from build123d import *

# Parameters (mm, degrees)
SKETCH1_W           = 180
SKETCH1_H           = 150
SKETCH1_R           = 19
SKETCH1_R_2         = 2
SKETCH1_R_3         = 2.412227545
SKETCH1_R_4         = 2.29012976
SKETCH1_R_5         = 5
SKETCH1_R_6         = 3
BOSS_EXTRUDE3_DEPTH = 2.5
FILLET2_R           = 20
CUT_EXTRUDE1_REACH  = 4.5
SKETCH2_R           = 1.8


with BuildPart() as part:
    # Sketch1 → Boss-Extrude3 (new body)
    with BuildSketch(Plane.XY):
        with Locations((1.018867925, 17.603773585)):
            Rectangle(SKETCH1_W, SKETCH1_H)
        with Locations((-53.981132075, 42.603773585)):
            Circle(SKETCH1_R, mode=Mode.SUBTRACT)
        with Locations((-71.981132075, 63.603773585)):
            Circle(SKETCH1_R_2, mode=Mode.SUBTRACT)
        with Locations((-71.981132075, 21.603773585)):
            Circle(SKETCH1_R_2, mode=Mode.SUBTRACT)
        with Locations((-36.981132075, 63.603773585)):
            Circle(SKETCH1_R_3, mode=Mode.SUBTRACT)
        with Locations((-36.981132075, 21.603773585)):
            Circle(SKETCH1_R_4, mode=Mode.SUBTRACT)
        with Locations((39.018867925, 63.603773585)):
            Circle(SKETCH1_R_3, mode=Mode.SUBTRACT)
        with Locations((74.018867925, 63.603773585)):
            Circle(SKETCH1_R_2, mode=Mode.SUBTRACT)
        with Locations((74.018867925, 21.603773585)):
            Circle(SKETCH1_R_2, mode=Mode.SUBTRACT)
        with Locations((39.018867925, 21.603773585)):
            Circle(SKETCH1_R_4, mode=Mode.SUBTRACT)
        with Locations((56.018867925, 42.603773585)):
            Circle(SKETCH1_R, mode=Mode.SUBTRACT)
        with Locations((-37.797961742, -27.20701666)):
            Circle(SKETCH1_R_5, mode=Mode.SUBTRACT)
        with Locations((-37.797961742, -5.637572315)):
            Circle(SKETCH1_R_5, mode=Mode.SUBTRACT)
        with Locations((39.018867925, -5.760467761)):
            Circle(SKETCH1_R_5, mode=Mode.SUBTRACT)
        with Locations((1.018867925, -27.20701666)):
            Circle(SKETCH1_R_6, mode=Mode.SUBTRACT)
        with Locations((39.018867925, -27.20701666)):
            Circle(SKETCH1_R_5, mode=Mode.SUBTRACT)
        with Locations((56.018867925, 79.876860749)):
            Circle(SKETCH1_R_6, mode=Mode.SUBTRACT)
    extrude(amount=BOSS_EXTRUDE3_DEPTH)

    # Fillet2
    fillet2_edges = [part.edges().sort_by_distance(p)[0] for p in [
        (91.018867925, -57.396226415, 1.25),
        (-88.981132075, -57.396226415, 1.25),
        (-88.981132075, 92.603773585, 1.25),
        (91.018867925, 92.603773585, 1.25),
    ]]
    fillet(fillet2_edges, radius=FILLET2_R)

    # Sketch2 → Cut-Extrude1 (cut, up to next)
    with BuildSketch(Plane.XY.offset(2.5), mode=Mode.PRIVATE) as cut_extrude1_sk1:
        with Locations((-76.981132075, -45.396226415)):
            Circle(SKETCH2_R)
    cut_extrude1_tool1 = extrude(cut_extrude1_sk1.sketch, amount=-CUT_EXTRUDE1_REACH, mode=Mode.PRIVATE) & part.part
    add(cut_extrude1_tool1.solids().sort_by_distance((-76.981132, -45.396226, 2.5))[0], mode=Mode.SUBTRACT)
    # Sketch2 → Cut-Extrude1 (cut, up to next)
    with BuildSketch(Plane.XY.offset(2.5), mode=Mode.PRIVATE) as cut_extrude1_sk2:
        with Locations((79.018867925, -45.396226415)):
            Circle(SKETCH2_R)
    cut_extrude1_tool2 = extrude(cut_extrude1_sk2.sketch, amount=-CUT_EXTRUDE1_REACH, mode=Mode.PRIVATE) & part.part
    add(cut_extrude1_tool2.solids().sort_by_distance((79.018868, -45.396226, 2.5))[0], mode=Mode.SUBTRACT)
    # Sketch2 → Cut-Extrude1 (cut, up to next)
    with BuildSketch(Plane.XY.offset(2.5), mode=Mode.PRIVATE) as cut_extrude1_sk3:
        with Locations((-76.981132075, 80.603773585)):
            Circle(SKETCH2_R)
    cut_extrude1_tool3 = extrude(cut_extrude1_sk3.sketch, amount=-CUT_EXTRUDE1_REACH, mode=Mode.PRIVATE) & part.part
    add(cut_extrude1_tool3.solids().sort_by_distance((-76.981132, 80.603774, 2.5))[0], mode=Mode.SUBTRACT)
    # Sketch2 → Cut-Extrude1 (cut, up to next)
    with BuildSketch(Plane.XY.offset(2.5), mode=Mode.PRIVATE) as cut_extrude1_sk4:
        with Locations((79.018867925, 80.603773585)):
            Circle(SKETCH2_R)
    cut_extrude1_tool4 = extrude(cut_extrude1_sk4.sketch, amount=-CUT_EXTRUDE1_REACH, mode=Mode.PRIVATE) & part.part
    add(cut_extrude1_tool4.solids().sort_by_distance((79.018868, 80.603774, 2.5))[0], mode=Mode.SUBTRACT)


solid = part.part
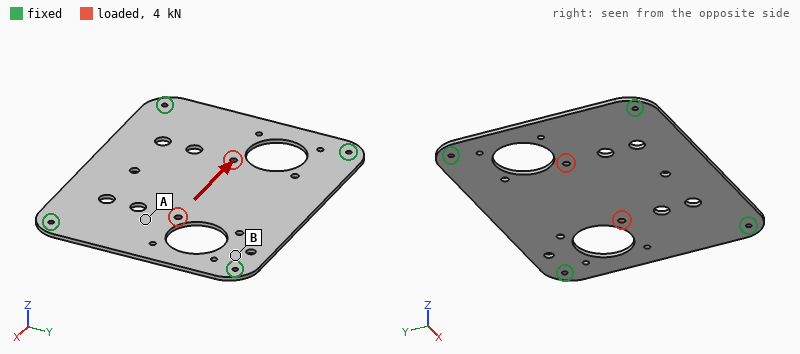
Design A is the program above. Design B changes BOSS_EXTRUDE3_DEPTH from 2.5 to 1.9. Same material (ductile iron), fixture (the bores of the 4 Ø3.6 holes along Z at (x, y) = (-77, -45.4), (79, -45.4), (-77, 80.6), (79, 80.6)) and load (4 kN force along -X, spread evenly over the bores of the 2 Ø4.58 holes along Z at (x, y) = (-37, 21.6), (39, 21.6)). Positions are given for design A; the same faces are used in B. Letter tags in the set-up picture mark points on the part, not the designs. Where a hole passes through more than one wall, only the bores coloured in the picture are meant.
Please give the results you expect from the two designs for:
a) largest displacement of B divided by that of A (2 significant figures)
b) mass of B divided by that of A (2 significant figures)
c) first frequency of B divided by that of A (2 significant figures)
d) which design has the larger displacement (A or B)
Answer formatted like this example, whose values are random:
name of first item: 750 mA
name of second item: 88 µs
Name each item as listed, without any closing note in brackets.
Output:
largest displacement of B divided by that of A: 1.3
mass of B divided by that of A: 0.76
first frequency of B divided by that of A: 0.77
which design has the larger displacement: B
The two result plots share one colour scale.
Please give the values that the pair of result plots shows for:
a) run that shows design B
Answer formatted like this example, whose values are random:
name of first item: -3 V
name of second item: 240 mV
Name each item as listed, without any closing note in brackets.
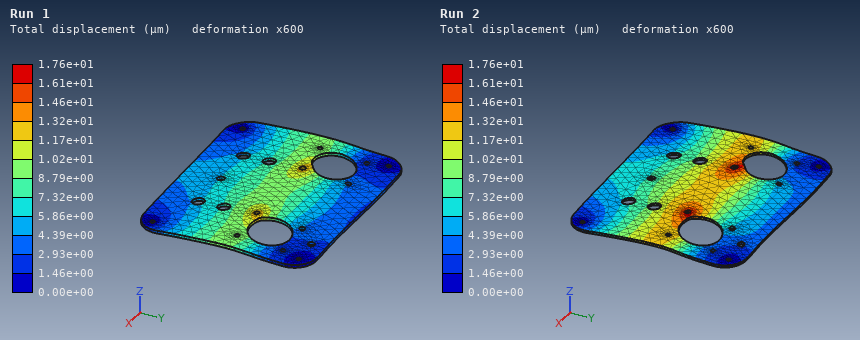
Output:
run that shows design B: Run 2
